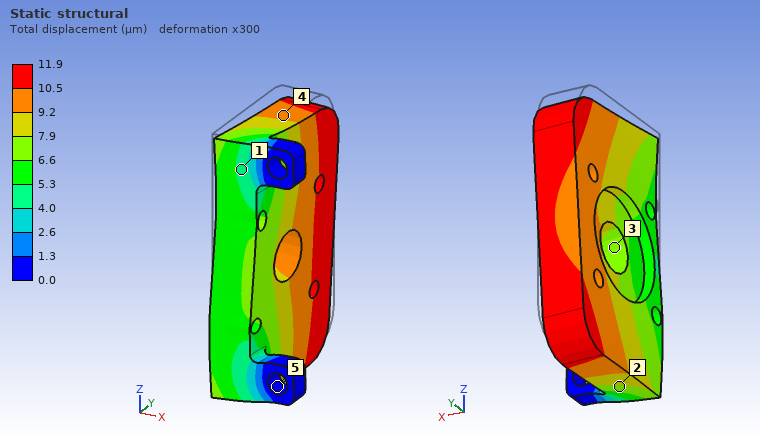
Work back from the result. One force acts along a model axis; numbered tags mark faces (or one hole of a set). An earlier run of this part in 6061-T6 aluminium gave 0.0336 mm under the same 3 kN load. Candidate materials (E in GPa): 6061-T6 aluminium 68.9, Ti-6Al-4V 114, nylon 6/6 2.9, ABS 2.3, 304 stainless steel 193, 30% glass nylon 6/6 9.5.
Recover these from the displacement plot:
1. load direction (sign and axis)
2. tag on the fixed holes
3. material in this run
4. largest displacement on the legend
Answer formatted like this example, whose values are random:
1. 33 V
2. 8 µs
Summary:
1. -Z
2. 5
3. 304 stainless steel
4. 11.9 µm
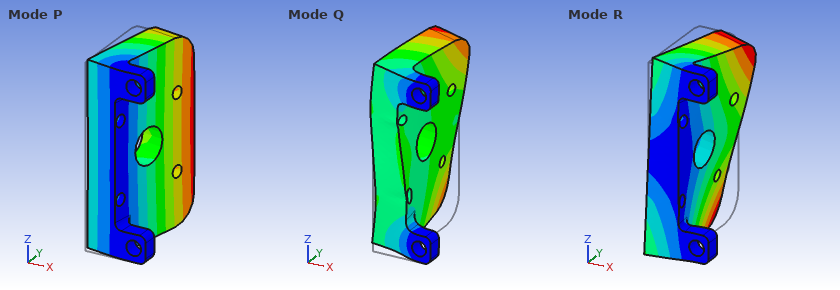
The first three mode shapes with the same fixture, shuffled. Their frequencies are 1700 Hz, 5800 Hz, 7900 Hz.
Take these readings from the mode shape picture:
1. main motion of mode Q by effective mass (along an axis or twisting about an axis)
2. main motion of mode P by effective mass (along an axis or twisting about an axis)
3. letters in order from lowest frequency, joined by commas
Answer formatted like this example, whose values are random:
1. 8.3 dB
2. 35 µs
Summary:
1. along Z
2. along X
3. P, R, Q
